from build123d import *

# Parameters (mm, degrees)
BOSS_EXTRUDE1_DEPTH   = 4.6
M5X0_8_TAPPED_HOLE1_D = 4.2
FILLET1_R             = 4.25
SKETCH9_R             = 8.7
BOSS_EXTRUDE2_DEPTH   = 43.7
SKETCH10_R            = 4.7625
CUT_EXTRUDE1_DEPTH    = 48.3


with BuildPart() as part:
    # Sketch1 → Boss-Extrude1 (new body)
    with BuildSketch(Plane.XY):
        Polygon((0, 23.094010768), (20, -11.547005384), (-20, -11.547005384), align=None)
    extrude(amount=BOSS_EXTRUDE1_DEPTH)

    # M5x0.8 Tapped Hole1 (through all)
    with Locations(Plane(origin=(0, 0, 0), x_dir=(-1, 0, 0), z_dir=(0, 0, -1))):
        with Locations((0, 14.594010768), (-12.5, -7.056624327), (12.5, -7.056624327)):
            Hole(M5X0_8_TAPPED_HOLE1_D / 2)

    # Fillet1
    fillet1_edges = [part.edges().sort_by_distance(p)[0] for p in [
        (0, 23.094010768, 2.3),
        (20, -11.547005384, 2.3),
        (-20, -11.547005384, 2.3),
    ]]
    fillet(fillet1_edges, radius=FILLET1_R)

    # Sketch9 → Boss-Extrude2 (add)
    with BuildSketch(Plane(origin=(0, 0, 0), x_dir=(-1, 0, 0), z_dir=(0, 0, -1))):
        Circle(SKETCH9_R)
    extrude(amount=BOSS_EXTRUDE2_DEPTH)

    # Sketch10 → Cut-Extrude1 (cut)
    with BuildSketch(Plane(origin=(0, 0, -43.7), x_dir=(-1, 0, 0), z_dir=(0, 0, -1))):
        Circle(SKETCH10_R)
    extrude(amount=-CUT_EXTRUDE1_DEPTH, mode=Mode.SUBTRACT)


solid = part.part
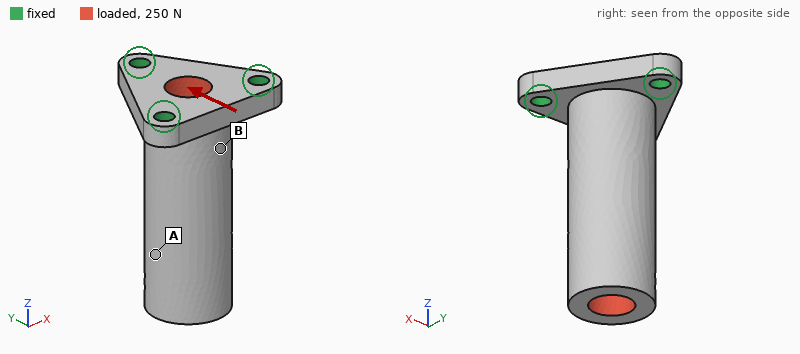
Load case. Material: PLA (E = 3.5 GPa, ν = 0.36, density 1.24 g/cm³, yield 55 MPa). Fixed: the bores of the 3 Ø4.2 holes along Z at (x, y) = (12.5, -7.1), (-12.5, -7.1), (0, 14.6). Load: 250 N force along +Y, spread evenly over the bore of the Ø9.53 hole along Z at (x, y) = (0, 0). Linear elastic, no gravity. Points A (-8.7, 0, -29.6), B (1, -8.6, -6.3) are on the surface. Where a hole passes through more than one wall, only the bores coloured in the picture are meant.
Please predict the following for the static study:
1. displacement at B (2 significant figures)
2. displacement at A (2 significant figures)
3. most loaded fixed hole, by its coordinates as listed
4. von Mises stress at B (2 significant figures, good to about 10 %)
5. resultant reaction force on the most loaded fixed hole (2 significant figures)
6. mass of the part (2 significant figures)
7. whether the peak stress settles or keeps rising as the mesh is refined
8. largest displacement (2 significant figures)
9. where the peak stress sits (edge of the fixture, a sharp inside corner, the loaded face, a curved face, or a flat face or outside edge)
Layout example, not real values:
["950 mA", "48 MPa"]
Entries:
["0.100 mm", "0.31 mm", "(0, 14.6)", "6.1 MPa", "310 N", "12 g", "keeps rising", "0.48 mm", "edge of the fixture"]
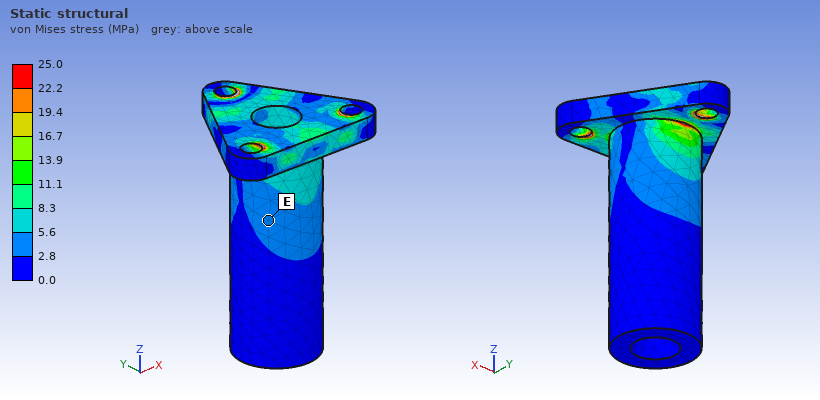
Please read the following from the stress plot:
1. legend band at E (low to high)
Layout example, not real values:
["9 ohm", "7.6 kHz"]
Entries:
["2.8 to 5.6 MPa"]
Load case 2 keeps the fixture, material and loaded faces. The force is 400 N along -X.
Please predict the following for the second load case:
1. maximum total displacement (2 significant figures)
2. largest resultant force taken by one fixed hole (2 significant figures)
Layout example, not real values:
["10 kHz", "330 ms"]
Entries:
["0.76 mm", "440 N"]
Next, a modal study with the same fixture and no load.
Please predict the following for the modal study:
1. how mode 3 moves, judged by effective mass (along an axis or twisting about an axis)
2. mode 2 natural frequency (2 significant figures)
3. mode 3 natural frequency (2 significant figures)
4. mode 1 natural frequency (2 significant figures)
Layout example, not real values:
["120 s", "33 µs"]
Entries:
["along Z", "1400 Hz", "5200 Hz", "1400 Hz"]
